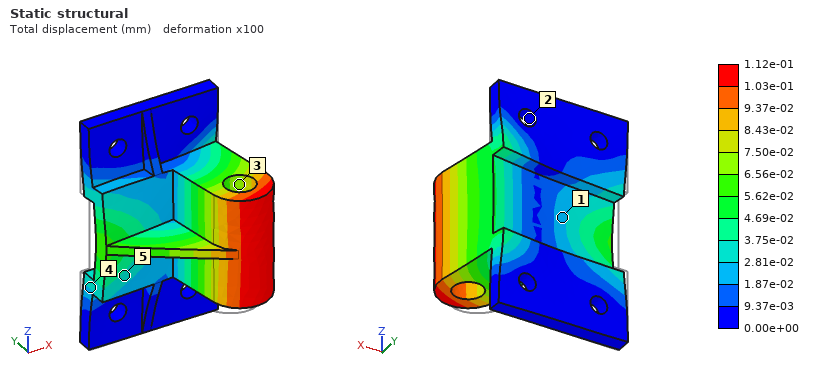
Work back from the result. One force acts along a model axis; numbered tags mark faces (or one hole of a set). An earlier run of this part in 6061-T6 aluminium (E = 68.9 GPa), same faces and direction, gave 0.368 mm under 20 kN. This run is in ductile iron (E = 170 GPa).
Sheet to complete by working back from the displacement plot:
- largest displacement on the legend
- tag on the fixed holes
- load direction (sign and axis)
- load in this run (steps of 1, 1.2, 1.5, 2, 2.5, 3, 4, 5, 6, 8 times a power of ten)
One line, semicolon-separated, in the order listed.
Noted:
1.12e-01 mm; 2; +X; 15 kN
